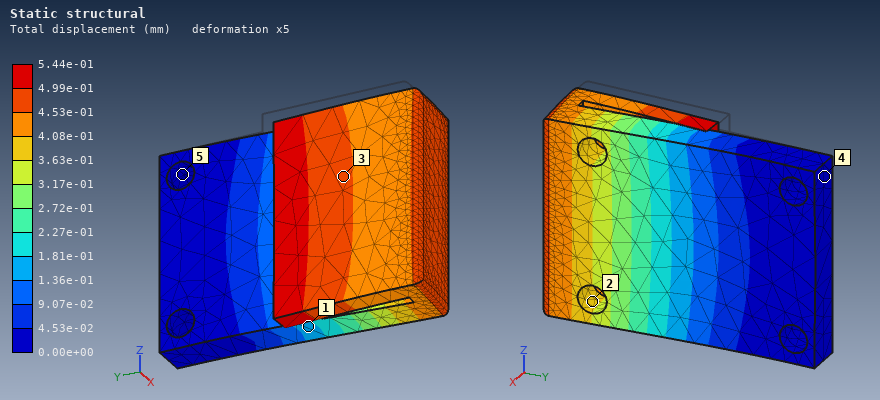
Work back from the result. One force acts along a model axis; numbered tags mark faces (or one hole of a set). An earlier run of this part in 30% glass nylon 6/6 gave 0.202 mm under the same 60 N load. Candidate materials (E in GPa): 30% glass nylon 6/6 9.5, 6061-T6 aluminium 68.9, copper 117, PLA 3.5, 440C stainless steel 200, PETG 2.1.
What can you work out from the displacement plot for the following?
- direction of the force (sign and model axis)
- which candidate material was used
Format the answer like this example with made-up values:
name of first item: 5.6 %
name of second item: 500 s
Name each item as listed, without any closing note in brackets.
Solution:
direction of the force: +X
which candidate material was used: PLA
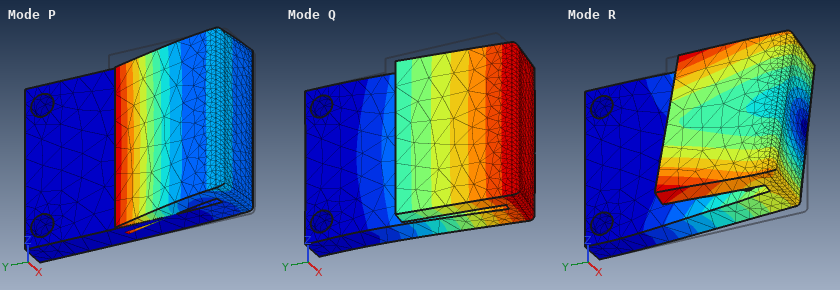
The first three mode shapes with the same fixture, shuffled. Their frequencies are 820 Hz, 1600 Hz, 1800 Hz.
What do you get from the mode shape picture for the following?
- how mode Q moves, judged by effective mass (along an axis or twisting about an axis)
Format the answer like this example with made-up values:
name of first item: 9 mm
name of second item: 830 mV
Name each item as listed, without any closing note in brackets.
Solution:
how mode Q moves, judged by effective mass: along X
